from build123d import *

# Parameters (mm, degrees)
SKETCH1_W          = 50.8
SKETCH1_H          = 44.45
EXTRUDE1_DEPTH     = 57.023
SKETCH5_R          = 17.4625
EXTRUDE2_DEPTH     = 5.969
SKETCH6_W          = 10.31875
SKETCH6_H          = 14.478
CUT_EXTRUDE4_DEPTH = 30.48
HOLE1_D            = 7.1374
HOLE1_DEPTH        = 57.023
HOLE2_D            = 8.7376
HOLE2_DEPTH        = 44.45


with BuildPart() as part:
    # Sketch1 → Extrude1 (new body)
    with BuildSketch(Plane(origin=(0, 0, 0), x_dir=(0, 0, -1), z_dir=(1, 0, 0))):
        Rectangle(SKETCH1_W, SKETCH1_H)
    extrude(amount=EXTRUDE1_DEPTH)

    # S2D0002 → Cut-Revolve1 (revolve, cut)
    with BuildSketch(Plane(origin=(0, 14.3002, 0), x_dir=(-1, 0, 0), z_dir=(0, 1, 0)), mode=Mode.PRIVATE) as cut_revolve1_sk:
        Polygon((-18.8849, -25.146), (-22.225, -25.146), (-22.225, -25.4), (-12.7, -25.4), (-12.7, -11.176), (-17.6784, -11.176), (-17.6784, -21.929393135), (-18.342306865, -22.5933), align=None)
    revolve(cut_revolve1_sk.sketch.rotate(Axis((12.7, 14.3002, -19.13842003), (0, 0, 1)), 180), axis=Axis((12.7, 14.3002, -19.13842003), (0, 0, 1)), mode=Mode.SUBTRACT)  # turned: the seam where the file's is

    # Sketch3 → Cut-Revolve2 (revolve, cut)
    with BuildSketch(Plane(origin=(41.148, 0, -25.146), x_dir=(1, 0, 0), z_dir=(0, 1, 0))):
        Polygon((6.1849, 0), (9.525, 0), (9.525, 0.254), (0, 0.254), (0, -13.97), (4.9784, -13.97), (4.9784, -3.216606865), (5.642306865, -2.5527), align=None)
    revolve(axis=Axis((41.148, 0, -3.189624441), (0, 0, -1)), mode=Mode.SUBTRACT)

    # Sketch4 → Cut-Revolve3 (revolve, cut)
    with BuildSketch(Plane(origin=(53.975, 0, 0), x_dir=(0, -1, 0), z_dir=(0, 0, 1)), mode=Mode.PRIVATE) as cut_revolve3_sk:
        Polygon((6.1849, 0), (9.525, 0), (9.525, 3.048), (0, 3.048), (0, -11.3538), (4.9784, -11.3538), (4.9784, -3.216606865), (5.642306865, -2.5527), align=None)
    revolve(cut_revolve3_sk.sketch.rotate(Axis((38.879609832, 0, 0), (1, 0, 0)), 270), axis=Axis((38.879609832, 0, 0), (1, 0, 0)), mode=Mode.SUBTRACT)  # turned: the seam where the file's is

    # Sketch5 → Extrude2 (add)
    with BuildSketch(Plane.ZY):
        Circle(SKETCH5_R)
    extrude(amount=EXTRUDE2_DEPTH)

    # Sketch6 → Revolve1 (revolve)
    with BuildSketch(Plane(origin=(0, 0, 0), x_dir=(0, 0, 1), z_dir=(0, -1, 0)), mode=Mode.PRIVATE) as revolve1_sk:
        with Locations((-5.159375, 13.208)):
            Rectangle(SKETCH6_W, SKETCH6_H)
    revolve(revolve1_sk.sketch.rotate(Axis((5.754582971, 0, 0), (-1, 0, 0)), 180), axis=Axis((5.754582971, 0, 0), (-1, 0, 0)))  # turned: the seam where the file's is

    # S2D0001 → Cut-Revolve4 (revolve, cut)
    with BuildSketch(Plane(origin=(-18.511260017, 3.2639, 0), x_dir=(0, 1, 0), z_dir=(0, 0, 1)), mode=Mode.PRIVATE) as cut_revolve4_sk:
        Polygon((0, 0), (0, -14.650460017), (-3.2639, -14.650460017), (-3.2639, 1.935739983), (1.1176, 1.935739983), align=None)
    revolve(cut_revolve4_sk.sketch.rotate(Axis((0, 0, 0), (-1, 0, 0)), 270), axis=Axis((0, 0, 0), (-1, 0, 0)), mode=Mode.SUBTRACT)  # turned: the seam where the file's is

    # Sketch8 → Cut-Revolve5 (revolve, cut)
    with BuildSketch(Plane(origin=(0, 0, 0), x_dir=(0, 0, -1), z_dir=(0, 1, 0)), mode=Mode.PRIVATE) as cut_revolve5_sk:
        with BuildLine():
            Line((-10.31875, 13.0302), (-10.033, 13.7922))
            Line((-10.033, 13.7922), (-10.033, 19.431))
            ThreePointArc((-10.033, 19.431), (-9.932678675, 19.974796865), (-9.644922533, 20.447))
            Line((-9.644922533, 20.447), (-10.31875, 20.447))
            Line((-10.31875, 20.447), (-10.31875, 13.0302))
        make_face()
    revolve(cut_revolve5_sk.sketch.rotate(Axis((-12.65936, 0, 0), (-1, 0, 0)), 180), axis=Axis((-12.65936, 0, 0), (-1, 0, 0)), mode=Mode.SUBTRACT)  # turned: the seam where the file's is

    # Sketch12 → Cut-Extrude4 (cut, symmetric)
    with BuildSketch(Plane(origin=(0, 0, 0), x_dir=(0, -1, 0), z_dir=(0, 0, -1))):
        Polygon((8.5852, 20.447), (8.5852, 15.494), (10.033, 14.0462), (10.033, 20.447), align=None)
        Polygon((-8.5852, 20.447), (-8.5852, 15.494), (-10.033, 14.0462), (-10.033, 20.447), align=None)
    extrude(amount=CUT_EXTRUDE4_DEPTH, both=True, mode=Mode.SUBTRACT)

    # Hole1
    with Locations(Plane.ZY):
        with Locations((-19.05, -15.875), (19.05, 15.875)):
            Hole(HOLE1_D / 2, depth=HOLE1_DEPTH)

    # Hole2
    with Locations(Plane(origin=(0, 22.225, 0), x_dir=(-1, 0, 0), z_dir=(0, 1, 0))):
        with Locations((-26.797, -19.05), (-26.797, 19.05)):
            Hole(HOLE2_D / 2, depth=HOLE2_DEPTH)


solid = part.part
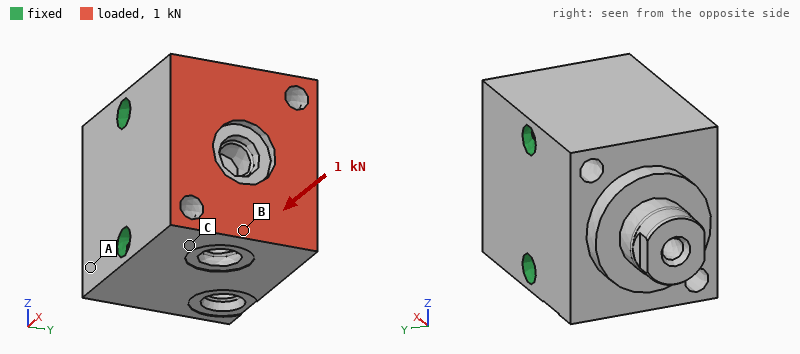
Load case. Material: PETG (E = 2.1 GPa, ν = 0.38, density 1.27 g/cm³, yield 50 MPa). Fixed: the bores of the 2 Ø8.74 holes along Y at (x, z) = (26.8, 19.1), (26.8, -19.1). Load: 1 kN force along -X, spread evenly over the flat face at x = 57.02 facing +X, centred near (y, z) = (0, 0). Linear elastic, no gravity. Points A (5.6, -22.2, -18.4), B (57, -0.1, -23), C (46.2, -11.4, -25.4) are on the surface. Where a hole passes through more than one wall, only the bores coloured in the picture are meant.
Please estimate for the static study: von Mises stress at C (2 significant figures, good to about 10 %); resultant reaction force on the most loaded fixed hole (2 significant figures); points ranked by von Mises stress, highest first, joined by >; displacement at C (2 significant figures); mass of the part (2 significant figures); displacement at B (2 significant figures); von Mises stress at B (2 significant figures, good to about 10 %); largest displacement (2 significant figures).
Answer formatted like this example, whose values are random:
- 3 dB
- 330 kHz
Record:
- 0.69 MPa
- 510 N
- C > B > A
- 6.3 µm
- 160 g
- 11 µm
- 0.43 MPa
- 11 µm
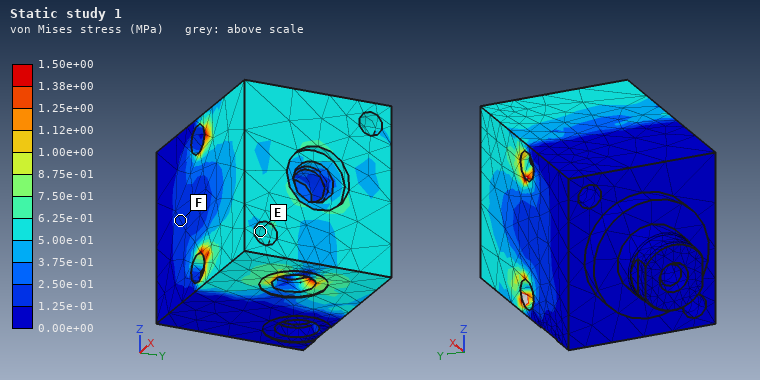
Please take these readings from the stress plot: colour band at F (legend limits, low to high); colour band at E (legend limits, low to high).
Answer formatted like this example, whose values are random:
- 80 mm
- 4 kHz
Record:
- 1.25e-01 to 2.50e-01 MPa
- 5.00e-01 to 6.25e-01 MPa
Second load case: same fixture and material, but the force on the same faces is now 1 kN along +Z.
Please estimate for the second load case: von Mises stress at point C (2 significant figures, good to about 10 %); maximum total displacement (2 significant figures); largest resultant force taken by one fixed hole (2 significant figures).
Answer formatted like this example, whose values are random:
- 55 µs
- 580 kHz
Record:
- 1.0 MPa
- 42 µm
- 860 N
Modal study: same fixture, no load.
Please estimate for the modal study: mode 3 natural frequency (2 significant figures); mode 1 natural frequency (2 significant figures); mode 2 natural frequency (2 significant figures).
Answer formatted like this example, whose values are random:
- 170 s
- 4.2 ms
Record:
- 4900 Hz
- 4000 Hz
- 4800 Hz
